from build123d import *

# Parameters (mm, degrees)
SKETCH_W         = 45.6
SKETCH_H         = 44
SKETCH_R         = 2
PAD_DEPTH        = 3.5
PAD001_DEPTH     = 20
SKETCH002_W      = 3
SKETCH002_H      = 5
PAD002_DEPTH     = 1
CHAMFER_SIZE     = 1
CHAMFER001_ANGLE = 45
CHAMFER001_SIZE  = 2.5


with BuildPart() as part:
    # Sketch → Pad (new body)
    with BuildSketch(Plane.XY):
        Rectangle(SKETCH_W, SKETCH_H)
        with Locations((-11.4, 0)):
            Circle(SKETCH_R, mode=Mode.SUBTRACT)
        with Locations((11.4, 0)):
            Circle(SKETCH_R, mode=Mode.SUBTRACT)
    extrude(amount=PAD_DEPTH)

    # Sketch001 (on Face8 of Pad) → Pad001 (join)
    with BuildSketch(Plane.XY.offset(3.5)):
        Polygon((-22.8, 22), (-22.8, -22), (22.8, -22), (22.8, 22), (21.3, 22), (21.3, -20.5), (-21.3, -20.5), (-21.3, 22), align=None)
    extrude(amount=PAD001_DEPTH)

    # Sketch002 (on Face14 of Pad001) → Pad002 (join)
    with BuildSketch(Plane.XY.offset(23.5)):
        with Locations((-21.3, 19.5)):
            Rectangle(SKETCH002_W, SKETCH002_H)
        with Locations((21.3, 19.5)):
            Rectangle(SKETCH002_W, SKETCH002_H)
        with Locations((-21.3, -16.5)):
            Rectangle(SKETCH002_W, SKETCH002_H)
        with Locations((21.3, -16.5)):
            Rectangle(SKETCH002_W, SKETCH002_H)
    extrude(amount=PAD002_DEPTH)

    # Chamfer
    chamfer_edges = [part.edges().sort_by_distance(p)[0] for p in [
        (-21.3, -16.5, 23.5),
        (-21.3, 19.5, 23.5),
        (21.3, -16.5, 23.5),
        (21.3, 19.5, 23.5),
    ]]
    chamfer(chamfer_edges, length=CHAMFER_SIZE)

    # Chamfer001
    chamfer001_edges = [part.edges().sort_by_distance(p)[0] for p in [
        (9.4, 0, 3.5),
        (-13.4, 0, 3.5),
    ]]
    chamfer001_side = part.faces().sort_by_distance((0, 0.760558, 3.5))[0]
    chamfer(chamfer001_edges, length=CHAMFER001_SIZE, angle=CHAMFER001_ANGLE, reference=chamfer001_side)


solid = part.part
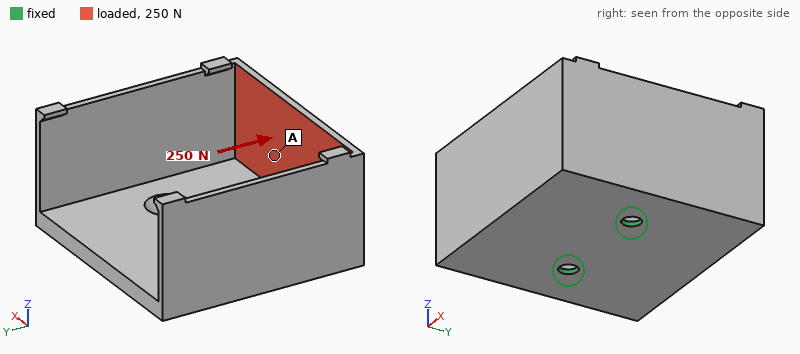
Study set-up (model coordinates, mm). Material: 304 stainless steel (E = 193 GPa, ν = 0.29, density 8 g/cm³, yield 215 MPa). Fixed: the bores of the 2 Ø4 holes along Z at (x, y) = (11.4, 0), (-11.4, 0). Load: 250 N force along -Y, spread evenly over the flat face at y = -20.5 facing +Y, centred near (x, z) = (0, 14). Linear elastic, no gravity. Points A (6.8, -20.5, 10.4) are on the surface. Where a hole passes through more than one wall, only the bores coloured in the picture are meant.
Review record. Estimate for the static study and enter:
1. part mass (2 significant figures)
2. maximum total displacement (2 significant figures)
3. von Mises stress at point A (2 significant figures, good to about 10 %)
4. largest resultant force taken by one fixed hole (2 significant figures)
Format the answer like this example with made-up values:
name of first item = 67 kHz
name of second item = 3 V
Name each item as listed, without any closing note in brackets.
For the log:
part mass = 86 g
maximum total displacement = 86 µm
von Mises stress at point A = 22 MPa
largest resultant force taken by one fixed hole = 130 N
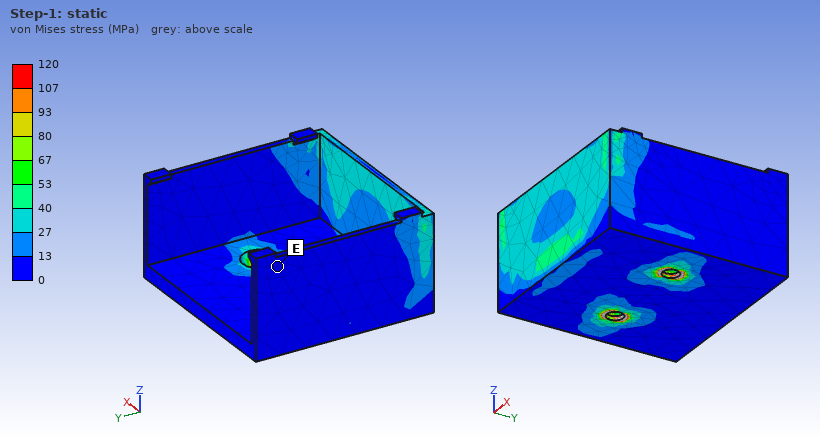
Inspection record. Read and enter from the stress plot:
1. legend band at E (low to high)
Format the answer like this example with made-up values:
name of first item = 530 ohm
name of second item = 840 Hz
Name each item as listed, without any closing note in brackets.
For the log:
legend band at E = 0 to 13 MPa
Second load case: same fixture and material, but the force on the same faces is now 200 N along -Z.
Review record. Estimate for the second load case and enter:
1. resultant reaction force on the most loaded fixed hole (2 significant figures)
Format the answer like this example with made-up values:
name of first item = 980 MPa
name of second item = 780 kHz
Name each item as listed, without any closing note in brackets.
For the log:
resultant reaction force on the most loaded fixed hole = 110 N
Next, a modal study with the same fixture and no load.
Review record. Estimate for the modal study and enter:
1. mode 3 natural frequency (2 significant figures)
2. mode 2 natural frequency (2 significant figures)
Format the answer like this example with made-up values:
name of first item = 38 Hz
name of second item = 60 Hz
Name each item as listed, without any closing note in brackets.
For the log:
mode 3 natural frequency = 2900 Hz
mode 2 natural frequency = 2700 Hz
